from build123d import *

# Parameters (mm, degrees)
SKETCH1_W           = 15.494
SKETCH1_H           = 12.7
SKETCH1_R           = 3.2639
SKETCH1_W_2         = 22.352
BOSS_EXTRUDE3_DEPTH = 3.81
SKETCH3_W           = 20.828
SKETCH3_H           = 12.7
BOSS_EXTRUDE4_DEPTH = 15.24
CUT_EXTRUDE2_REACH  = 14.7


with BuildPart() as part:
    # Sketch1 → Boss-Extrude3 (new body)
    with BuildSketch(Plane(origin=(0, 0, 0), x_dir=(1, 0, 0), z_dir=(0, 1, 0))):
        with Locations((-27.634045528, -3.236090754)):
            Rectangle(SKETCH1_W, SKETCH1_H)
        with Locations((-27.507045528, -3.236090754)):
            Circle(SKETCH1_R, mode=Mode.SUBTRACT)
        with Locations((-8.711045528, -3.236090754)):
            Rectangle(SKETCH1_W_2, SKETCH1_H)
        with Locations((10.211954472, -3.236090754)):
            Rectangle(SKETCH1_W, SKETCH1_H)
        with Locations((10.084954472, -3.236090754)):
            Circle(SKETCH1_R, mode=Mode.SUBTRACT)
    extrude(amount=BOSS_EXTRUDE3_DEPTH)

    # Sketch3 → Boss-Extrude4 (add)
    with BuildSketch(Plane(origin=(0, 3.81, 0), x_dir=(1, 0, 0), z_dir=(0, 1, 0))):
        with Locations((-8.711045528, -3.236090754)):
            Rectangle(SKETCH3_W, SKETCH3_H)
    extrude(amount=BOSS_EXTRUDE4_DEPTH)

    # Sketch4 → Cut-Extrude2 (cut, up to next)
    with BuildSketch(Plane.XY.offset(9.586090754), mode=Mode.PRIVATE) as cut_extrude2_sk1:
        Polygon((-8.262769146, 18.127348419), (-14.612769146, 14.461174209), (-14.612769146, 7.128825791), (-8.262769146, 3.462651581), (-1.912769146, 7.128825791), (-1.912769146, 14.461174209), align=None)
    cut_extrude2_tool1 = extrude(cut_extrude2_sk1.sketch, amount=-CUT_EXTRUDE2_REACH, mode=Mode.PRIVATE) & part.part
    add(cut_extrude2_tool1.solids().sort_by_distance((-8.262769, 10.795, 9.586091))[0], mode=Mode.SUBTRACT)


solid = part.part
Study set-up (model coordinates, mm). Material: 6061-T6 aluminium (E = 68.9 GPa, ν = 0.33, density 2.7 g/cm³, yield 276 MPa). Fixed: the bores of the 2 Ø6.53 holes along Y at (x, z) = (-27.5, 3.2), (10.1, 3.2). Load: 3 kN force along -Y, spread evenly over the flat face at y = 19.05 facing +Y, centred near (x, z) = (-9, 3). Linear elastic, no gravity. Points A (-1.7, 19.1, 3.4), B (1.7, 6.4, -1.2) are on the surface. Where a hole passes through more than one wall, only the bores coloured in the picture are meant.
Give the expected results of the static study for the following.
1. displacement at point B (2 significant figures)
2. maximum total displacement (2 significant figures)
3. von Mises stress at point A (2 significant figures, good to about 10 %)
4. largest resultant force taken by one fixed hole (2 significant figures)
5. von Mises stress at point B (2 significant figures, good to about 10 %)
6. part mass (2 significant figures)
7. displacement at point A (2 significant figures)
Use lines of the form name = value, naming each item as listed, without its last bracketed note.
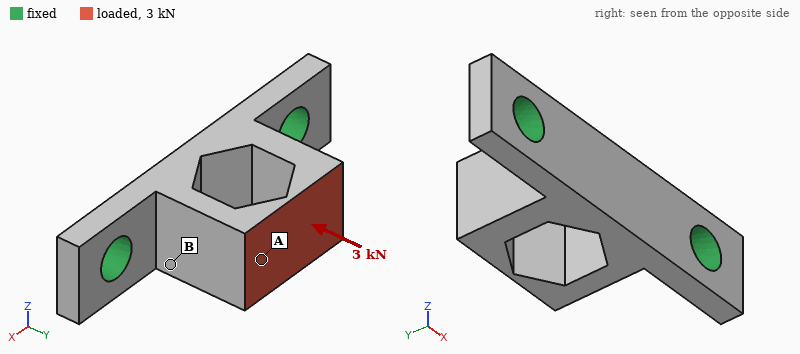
displacement at point B = 29 µm
maximum total displacement = 48 µm
von Mises stress at point A = 31 MPa
largest resultant force taken by one fixed hole = 1.6 kN
von Mises stress at point B = 92 MPa
part mass = 12 g
displacement at point A = 35 µm
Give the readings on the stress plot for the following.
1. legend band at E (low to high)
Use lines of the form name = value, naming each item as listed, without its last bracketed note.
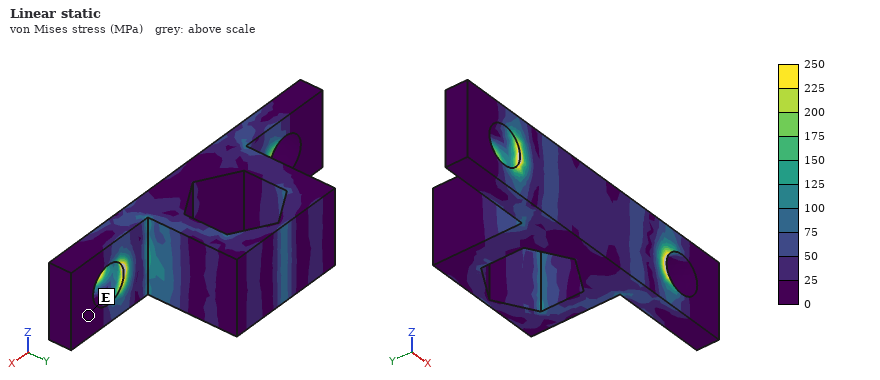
legend band at E = 0 to 25 MPa
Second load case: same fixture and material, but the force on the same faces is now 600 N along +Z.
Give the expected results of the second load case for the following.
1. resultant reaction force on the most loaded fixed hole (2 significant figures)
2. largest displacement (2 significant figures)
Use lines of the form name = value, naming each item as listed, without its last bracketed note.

resultant reaction force on the most loaded fixed hole = 300 N
largest displacement = 0.11 mm
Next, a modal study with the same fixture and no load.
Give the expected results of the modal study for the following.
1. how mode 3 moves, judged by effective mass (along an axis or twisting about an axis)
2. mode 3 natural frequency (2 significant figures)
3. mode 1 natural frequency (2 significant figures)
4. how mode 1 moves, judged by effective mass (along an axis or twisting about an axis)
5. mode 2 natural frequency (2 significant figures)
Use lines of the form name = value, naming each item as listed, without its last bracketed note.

how mode 3 moves, judged by effective mass = along Y
mode 3 natural frequency = 15 kHz
mode 1 natural frequency = 7100 Hz
how mode 1 moves, judged by effective mass = along Z
mode 2 natural frequency = 14 kHz
